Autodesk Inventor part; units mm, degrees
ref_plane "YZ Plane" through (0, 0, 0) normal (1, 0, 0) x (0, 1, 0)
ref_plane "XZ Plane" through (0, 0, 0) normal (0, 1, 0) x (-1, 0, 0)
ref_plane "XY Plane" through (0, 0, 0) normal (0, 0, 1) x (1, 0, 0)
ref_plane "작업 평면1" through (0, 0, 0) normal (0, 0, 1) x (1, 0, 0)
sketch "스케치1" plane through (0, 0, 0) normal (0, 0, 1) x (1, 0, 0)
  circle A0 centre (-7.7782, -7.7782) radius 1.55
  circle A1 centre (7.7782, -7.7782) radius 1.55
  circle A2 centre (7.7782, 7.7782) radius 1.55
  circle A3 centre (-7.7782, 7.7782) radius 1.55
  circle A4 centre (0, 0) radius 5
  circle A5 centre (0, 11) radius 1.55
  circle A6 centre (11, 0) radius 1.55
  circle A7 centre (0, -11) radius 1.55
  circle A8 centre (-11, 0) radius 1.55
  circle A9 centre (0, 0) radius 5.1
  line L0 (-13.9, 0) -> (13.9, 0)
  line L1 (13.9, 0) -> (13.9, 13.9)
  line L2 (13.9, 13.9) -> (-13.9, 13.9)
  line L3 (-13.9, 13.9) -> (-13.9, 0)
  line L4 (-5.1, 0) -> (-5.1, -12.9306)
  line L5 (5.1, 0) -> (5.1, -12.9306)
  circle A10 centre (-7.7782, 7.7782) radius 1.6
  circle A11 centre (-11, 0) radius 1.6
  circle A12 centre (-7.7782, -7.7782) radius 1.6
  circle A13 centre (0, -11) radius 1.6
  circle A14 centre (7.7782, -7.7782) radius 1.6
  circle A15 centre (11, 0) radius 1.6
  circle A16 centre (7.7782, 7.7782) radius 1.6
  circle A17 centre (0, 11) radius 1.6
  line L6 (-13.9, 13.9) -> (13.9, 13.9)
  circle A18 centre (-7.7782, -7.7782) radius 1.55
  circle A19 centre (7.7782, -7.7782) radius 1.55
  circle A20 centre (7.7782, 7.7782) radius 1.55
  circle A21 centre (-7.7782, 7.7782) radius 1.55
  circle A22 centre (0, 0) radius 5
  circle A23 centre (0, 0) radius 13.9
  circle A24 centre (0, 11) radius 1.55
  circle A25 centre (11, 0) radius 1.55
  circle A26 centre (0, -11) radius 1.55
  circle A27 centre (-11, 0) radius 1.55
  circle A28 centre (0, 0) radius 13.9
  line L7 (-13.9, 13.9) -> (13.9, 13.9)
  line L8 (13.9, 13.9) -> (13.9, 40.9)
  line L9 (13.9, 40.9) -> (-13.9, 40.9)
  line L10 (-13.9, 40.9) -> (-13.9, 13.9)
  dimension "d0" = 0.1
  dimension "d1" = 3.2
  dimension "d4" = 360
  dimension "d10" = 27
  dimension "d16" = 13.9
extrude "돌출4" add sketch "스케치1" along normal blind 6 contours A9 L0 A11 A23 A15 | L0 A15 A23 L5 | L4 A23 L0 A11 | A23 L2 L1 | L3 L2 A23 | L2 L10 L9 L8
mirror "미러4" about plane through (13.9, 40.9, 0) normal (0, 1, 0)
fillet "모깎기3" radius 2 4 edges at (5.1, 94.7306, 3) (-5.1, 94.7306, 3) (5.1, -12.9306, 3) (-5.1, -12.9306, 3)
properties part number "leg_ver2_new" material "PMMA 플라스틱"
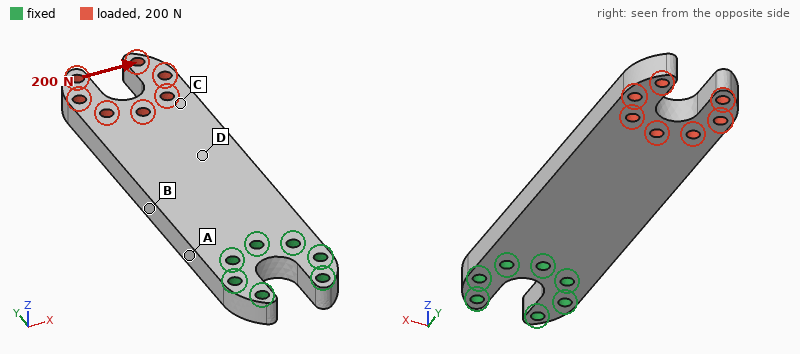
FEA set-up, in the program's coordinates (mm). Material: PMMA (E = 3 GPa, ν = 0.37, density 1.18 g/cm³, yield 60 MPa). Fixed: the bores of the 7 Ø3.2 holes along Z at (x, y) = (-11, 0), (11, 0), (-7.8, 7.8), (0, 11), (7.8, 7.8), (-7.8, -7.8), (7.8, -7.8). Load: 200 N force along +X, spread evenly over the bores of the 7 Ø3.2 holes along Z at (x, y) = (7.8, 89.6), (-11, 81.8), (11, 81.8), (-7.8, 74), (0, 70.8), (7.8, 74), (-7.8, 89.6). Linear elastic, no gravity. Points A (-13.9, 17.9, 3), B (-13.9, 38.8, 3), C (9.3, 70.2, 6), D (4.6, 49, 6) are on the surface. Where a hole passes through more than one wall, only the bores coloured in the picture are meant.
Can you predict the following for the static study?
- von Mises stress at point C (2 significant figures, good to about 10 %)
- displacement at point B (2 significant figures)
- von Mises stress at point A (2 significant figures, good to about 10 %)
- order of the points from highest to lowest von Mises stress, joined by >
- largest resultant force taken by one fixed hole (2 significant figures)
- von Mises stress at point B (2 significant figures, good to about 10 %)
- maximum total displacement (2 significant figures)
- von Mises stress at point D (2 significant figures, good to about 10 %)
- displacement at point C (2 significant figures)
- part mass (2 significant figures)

1.7 MPa
0.30 mm
16 MPa
A > B > D > C
560 N
11 MPa
1.2 mm
3.9 MPa
0.76 mm
17 g
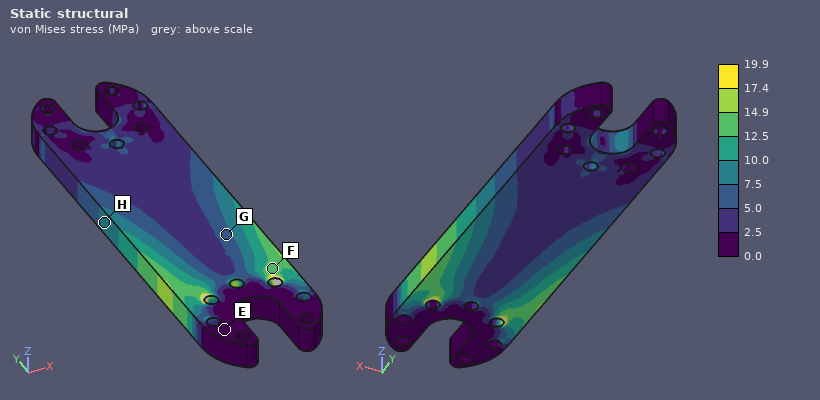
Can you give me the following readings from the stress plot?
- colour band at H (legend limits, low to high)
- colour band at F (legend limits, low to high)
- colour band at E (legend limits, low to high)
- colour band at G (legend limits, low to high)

7.5 to 10.0 MPa
12.5 to 14.9 MPa
0.0 to 2.5 MPa
5.0 to 7.5 MPa
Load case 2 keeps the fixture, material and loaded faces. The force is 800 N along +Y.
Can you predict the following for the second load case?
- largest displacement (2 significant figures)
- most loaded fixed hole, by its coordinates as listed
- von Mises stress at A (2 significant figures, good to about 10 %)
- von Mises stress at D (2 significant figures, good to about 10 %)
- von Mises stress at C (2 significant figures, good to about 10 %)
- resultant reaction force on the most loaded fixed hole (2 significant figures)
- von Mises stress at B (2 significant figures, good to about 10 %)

0.14 mm
(0, 11)
3.7 MPa
4.8 MPa
5.7 MPa
280 N
4.8 MPa
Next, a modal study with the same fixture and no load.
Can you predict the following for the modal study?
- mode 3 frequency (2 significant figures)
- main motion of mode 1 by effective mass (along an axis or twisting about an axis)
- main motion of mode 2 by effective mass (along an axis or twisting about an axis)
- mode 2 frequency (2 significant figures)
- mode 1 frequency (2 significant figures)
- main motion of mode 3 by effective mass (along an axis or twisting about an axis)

1300 Hz
along Z
along X
1100 Hz
280 Hz
twisting about Y
